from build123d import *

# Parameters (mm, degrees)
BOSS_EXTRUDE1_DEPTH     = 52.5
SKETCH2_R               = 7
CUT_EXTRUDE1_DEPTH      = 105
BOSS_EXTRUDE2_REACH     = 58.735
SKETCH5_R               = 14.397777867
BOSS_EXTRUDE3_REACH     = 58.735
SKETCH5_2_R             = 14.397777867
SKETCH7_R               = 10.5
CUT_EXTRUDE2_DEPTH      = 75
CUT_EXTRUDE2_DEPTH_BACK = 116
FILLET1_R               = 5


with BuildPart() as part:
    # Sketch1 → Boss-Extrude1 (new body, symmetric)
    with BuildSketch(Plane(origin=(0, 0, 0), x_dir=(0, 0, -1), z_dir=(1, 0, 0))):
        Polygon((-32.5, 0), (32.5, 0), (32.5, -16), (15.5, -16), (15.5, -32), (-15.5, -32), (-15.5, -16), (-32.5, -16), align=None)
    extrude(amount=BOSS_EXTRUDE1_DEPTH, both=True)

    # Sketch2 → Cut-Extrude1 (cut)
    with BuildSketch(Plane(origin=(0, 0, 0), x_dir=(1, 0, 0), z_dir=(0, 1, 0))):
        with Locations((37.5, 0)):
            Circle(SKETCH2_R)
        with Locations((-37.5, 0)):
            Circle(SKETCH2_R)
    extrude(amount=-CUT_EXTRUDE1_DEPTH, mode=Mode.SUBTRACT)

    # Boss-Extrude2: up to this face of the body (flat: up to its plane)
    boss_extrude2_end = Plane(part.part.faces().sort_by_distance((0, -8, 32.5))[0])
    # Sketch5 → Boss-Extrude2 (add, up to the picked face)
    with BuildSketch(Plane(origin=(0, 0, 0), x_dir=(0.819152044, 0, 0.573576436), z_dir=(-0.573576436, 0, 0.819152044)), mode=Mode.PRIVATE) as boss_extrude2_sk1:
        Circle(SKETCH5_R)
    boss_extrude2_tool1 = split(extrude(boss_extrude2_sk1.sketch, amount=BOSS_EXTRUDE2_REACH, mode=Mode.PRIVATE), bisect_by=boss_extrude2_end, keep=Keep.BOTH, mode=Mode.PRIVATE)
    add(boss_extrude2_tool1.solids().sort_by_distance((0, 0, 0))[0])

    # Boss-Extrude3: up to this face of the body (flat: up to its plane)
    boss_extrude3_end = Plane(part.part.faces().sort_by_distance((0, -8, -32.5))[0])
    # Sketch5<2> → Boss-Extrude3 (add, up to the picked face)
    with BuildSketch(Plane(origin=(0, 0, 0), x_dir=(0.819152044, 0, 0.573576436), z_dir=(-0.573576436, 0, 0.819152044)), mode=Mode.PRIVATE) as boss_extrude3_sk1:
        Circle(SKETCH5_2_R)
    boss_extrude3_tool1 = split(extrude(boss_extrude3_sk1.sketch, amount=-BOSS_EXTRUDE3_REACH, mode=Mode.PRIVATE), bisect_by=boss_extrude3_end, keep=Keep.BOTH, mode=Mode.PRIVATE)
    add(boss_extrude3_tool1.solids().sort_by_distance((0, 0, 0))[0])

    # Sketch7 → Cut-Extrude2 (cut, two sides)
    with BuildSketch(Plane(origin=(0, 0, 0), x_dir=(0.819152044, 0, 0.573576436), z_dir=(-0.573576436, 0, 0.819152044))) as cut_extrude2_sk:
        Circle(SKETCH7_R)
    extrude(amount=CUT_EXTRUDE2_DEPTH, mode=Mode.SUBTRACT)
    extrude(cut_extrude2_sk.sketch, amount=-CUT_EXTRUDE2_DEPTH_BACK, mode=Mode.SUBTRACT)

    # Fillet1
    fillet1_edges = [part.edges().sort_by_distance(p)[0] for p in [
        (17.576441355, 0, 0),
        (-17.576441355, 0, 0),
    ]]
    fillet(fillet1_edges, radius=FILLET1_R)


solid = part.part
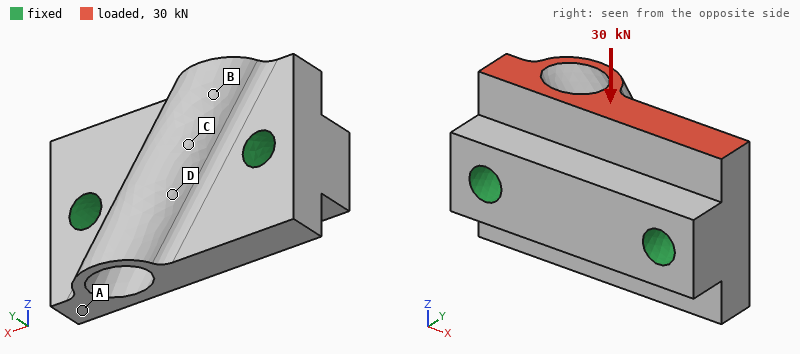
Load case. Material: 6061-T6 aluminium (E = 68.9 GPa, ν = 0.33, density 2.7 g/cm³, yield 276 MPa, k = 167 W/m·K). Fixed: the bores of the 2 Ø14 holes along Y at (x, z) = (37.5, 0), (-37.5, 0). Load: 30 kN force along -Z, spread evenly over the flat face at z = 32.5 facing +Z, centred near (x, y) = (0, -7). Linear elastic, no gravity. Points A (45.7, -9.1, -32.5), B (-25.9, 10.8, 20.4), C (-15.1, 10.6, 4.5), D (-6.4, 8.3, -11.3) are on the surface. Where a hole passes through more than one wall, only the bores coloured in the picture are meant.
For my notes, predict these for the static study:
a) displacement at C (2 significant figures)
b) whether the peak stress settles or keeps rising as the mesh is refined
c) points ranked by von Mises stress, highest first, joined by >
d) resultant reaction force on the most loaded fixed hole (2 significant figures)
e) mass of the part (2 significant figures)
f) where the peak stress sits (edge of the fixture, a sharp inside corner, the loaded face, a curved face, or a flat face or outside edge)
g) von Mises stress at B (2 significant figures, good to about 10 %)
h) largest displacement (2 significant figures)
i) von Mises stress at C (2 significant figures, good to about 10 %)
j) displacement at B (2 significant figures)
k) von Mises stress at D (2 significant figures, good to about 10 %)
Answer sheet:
20 µm
keeps rising
B > C > D > A
15 kN
410 g
a sharp inside corner
32 MPa
52 µm
22 MPa
29 µm
13 MPa
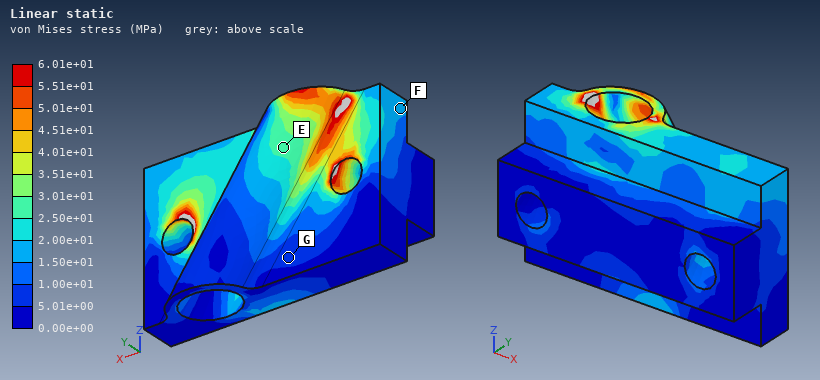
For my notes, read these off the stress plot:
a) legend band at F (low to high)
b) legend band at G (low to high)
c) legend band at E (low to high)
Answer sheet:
1.50e+01 to 2.00e+01 MPa
5.01e+00 to 1.00e+01 MPa
2.50e+01 to 3.01e+01 MPa
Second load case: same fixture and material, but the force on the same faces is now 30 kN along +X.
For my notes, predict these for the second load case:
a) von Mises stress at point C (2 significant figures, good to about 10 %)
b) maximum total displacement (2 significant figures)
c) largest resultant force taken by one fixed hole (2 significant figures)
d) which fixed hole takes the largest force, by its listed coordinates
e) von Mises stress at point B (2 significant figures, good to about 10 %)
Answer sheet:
16 MPa
67 µm
20 kN
(37.5, 0)
28 MPa
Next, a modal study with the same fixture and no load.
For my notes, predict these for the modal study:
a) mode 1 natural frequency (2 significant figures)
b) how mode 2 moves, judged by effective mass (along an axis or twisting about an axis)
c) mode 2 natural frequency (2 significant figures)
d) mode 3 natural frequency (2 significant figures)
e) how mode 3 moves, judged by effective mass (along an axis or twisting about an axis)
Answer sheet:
11 kHz
along Y
14 kHz
15 kHz
along Z
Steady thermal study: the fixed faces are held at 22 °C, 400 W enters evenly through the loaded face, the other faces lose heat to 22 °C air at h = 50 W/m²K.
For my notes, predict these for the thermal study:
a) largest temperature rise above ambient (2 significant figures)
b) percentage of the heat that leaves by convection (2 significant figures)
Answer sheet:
55 K
4.0 %
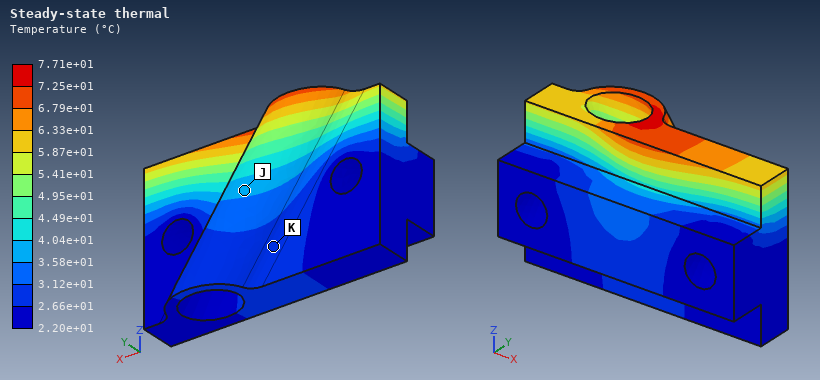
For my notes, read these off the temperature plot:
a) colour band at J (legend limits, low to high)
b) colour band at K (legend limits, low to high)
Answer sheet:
3.58e+01 to 4.04e+01 °C
2.66e+01 to 3.12e+01 °C
